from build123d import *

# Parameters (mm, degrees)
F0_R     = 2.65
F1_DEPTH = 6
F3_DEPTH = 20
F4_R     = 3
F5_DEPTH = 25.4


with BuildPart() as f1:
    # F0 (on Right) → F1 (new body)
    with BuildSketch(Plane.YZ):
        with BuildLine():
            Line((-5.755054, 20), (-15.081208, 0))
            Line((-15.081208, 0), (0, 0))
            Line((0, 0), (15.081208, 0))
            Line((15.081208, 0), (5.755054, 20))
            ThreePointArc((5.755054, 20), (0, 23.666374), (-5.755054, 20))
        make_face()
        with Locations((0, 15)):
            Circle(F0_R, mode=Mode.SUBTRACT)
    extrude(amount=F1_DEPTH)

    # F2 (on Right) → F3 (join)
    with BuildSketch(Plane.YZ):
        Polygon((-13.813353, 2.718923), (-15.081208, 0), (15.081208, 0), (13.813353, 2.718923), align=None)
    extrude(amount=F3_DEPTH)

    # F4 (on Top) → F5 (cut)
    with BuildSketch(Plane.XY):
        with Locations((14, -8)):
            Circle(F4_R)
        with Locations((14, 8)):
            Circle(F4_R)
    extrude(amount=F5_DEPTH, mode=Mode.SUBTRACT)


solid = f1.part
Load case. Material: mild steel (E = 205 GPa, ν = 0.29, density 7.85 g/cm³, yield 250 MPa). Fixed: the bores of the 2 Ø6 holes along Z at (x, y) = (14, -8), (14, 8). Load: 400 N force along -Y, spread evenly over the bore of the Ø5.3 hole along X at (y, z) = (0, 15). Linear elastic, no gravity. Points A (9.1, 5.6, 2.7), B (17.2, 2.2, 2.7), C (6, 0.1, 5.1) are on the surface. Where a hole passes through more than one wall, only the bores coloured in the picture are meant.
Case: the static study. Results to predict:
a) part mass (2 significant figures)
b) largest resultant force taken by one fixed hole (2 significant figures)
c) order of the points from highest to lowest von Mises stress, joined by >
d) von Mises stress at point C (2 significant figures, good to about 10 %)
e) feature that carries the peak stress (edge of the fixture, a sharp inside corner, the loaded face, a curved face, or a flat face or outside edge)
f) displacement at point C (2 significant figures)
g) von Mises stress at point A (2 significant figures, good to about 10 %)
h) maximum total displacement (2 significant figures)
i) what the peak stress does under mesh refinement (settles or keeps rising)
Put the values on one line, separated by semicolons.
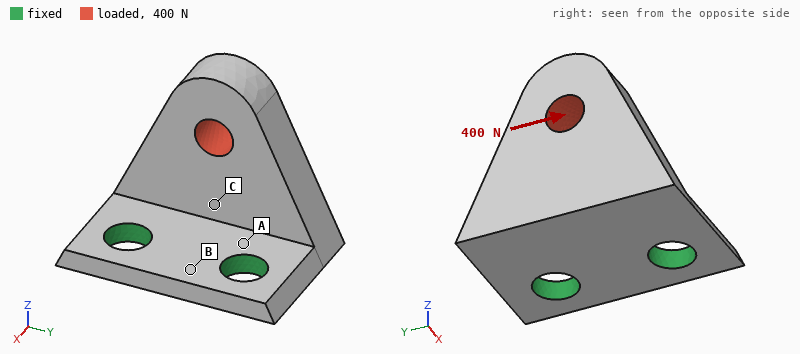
27 g; 400 N; A > C > B; 21 MPa; edge of the fixture; 2.4 µm; 35 MPa; 12 µm; keeps rising
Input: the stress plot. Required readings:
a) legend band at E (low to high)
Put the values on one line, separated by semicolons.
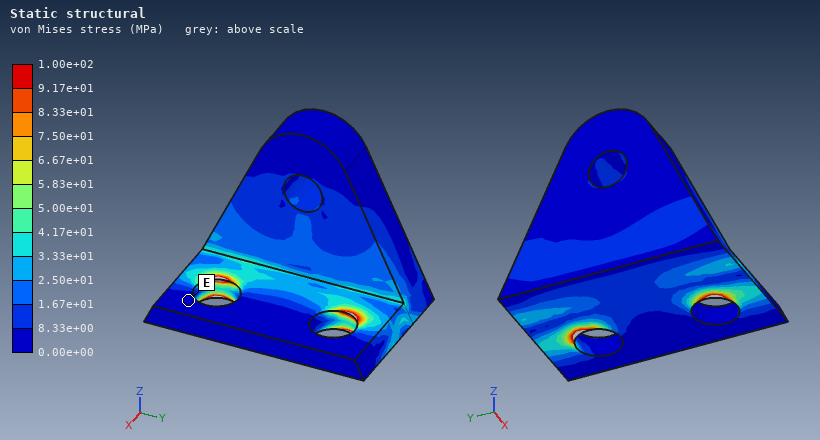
0.00e+00 to 8.33e+00 MPa
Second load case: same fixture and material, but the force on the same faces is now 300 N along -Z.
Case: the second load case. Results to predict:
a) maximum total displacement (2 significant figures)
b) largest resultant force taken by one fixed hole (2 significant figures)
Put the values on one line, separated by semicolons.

28 µm; 150 N
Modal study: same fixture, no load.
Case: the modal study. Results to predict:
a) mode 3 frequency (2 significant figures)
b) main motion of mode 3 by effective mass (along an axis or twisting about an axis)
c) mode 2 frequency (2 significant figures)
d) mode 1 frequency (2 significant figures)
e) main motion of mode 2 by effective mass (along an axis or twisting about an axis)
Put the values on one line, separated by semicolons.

16 kHz; along Z; 9800 Hz; 3600 Hz; along Y
